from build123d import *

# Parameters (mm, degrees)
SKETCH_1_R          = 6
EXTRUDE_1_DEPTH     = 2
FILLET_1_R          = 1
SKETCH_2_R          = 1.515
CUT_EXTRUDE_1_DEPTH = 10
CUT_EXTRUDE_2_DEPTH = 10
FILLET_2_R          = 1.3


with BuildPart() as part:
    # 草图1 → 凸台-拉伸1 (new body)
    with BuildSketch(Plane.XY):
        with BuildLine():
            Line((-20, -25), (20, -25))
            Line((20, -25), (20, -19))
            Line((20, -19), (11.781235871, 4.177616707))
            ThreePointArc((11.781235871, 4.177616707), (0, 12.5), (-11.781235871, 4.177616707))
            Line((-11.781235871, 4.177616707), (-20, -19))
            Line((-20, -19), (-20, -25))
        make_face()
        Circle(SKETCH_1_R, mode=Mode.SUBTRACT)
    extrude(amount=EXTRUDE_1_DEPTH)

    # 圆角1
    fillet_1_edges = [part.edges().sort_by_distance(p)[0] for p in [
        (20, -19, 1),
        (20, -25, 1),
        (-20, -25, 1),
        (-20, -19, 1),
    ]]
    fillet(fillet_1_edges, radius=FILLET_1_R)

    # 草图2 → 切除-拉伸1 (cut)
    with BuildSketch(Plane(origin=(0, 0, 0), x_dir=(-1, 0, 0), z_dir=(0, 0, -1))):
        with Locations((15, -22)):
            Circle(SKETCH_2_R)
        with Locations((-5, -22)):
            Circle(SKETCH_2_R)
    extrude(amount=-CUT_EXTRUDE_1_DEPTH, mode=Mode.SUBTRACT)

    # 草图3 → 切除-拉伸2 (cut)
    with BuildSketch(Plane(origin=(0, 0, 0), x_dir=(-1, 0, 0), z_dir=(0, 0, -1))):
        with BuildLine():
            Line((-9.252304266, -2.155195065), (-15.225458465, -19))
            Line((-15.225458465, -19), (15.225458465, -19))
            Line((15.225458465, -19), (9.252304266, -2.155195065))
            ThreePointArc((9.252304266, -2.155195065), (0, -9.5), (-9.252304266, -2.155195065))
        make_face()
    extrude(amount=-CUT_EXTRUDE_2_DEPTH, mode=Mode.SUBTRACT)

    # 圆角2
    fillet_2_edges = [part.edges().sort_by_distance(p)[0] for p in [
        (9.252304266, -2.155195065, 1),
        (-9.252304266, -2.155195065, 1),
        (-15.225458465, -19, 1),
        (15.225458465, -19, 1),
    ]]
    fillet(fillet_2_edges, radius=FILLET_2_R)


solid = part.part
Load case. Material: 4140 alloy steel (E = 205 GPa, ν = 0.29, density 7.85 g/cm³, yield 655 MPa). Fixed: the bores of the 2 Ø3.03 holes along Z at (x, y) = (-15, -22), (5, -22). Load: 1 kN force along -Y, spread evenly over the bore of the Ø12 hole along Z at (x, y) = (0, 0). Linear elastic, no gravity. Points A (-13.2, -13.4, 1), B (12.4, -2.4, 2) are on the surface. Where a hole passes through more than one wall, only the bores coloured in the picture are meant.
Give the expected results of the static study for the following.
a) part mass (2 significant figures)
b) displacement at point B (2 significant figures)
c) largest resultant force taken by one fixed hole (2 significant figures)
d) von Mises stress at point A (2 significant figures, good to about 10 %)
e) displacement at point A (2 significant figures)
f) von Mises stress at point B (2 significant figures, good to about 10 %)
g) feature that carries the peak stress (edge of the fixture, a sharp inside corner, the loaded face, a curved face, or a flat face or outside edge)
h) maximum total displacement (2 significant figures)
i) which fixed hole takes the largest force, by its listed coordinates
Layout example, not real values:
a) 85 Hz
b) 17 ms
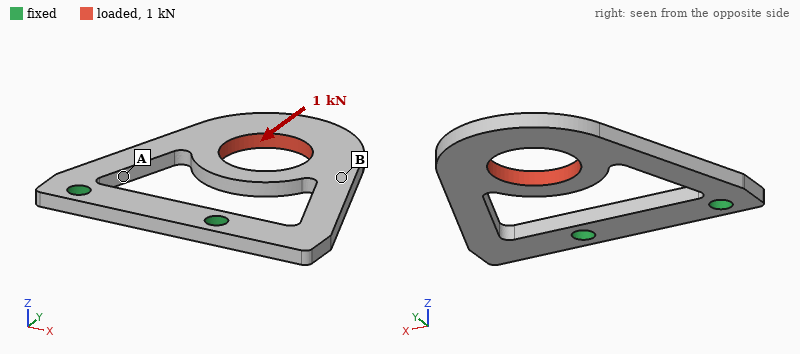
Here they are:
a) 11 g
b) 48 µm
c) 550 N
d) 140 MPa
e) 9.3 µm
f) 69 MPa
g) edge of the fixture
h) 54 µm
i) (5, -22)
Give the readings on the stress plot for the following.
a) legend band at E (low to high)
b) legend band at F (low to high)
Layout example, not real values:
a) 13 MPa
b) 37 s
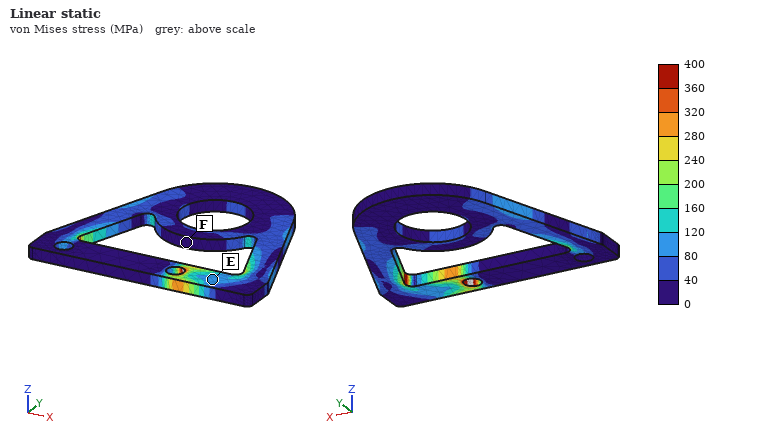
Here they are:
a) 80 to 120 MPa
b) 0 to 40 MPa
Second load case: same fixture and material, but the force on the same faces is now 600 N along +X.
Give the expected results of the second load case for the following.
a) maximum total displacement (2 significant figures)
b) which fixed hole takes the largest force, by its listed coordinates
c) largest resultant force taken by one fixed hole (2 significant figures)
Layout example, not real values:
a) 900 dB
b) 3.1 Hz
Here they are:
a) 88 µm
b) (-15, -22)
c) 470 N
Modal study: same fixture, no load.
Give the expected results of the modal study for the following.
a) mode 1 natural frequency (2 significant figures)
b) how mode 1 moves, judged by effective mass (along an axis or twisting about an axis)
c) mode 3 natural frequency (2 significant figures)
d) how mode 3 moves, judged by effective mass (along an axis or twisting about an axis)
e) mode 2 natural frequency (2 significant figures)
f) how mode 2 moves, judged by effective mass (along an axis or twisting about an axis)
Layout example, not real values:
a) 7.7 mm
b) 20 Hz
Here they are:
a) 980 Hz
b) along Z
c) 5300 Hz
d) along X
e) 3500 Hz
f) twisting about Y
